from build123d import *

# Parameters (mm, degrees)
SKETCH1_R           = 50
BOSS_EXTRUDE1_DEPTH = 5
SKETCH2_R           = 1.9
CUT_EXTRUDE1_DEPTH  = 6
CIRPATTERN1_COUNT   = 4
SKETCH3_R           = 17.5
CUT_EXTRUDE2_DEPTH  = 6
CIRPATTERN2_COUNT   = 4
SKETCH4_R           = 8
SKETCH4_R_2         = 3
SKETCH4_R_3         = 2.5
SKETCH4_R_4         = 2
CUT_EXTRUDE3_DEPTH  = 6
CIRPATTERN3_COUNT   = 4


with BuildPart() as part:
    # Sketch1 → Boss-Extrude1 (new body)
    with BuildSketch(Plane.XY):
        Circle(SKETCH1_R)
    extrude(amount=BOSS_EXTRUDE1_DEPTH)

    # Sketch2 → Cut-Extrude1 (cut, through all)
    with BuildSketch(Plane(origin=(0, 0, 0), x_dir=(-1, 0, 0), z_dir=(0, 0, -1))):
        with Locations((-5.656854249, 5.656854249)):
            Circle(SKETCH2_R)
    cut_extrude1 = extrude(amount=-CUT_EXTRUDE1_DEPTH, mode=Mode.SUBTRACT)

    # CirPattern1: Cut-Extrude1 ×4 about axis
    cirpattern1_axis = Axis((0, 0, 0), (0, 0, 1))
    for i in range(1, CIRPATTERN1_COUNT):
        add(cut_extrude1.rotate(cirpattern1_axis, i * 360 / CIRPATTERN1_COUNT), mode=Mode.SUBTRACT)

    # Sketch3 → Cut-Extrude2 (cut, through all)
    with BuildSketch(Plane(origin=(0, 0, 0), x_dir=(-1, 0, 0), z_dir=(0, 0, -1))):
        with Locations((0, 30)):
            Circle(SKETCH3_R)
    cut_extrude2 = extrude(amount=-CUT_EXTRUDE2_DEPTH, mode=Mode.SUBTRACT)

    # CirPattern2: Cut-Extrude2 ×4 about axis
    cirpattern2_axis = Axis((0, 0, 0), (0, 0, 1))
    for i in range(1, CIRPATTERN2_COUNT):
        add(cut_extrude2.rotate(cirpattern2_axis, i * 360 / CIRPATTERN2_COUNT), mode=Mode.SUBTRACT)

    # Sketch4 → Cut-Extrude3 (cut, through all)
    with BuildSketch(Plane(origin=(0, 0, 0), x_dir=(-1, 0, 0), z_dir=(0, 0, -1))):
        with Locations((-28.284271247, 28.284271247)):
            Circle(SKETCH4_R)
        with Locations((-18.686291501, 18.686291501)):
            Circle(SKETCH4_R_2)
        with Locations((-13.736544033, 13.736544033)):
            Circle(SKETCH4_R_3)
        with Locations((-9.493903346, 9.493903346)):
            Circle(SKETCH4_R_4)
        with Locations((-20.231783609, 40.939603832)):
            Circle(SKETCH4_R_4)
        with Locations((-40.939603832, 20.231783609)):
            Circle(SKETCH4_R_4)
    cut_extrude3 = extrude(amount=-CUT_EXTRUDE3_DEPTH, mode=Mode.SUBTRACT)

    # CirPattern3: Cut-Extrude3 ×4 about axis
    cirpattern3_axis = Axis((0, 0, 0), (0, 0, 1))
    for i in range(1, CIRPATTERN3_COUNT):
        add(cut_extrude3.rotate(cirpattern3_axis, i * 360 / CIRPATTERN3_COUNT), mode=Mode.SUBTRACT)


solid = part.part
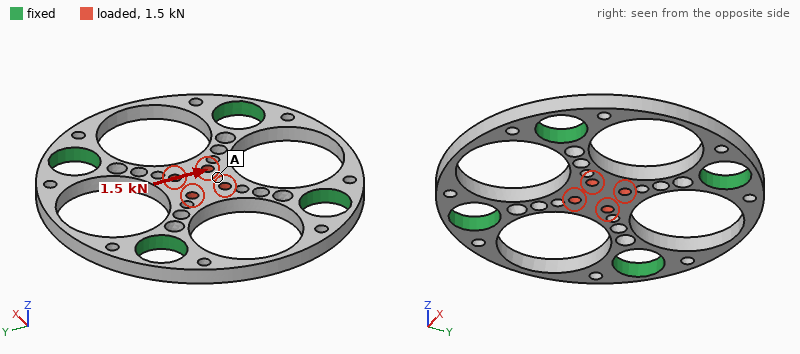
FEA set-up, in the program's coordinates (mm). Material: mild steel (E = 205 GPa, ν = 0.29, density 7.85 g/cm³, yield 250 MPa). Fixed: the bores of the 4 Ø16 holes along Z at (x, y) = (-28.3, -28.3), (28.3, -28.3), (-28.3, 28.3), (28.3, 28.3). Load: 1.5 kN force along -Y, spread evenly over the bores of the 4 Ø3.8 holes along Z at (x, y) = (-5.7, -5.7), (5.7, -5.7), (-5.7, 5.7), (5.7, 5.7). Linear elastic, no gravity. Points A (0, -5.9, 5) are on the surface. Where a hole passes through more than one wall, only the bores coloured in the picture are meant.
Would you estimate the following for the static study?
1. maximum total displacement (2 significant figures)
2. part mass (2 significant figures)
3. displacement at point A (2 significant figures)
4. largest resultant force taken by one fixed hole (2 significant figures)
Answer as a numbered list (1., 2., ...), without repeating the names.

1. 3.8 µm
2. 110 g
3. 3.8 µm
4. 480 N
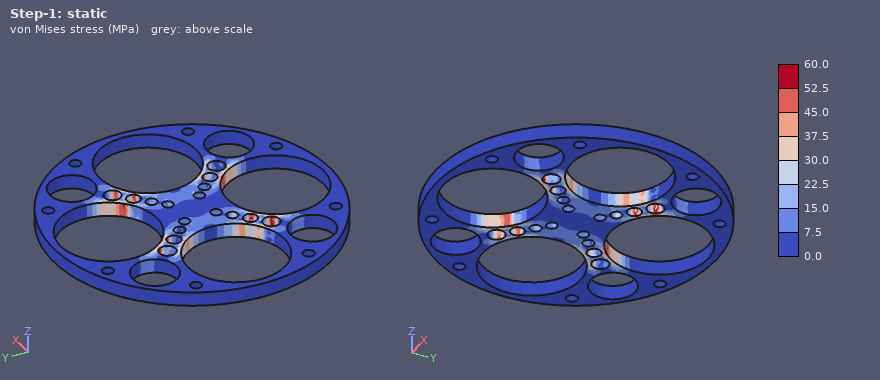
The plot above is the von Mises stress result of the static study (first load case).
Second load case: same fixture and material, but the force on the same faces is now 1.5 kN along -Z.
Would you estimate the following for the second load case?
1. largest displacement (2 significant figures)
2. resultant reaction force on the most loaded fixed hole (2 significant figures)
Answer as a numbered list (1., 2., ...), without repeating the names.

1. 47 µm
2. 380 N
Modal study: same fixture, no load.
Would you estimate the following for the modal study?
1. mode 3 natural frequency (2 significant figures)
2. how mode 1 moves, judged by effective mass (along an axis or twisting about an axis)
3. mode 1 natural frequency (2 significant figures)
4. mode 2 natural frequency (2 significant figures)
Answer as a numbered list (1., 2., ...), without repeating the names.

1. 9200 Hz
2. along Z
3. 6200 Hz
4. 9200 Hz
